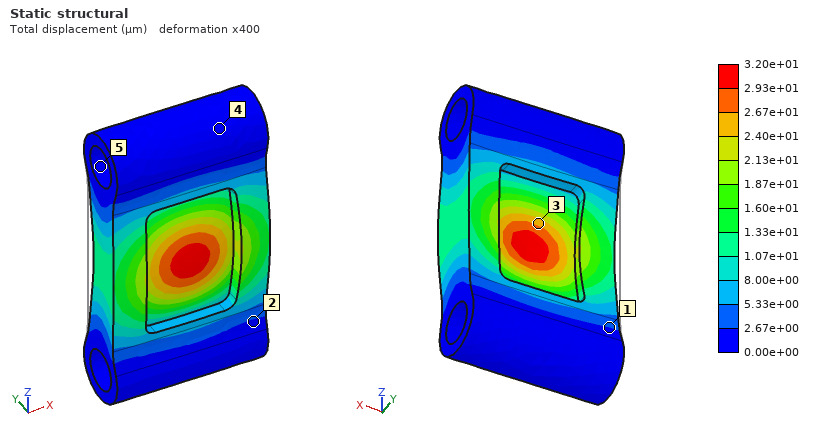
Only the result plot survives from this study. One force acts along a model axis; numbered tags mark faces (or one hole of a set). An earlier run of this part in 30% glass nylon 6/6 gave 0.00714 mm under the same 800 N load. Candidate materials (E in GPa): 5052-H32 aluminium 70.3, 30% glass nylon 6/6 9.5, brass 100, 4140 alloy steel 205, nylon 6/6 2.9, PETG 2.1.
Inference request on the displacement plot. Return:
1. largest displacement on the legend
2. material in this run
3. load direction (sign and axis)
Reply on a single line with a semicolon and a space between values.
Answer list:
3.20e+01 µm; PETG; -Y
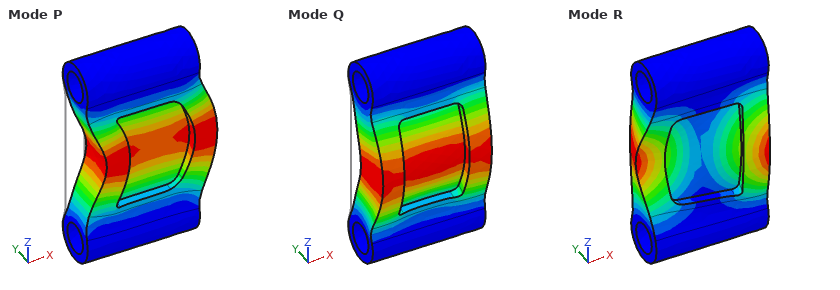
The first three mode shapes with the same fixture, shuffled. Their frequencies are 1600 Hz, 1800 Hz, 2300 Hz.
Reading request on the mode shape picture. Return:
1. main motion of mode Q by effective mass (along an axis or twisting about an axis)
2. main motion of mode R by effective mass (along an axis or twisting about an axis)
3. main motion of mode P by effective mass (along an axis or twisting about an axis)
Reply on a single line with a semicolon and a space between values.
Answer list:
along Y; twisting about Z; along X
